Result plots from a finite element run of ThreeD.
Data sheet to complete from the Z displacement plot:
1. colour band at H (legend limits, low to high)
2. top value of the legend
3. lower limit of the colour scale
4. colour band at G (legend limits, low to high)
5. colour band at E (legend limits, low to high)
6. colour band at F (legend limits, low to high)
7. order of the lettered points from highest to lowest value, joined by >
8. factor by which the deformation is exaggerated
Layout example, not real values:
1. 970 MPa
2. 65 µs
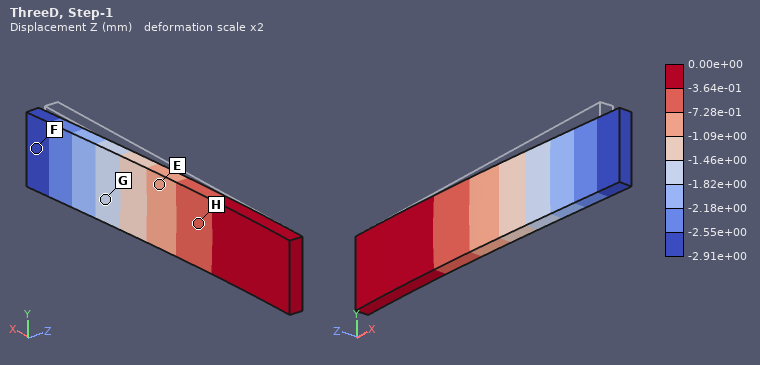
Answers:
1. -7.28e-01 to -3.64e-01 mm
2. 0.00e+00 mm
3. -2.91e+00 mm
4. -1.82e+00 to -1.46e+00 mm
5. -1.09e+00 to -7.28e-01 mm
6. -2.91e+00 to -2.55e+00 mm
7. H > E > G > F
8. 2
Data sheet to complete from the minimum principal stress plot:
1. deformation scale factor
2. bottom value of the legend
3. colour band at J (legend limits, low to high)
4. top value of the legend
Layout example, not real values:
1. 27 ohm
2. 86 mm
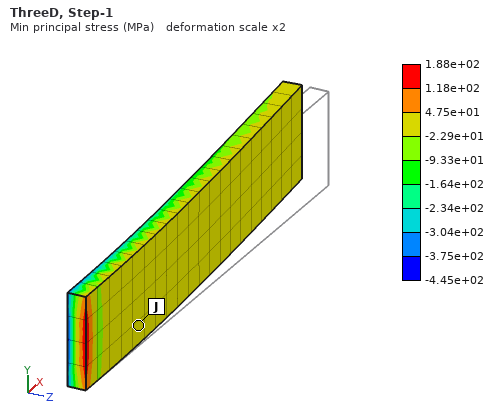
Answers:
1. 2
2. -4.45e+02 MPa
3. -2.29e+01 to 4.75e+01 MPa
4. 1.88e+02 MPa
